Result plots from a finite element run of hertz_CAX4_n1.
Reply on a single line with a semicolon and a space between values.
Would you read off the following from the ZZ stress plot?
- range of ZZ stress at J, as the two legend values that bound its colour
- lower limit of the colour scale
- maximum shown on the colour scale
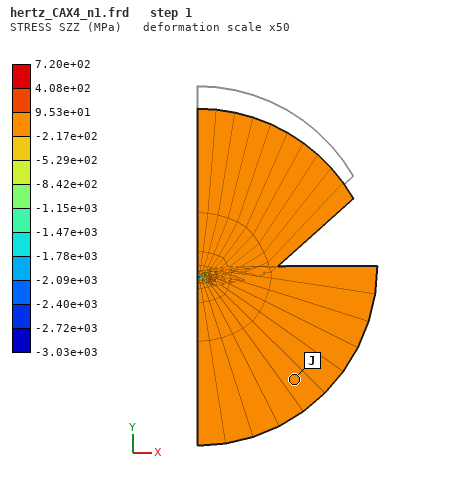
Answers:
-2.17e+02 to 9.53e+01 MPa; -3.03e+03 MPa; 7.20e+02 MPa
